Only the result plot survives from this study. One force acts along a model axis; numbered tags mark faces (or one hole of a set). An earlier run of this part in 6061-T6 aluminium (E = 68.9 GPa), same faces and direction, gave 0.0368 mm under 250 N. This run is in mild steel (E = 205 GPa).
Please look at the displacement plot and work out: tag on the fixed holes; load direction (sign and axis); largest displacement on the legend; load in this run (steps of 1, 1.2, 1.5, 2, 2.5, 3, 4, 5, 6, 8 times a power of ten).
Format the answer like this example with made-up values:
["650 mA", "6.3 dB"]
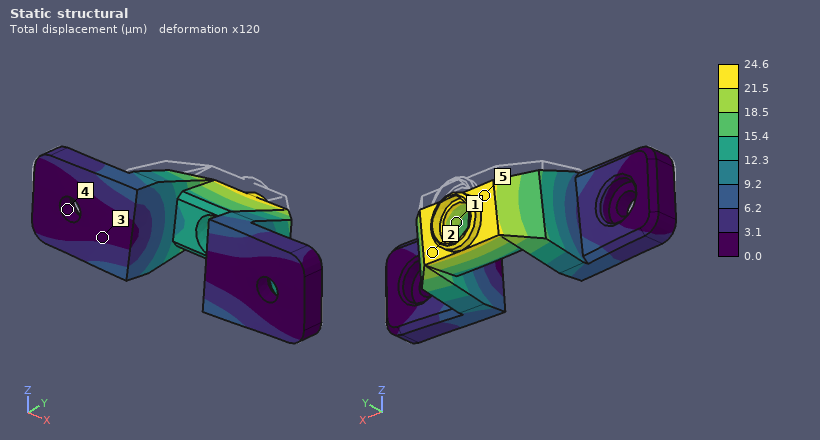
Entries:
["4", "-Z", "24.6 µm", "500 N"]
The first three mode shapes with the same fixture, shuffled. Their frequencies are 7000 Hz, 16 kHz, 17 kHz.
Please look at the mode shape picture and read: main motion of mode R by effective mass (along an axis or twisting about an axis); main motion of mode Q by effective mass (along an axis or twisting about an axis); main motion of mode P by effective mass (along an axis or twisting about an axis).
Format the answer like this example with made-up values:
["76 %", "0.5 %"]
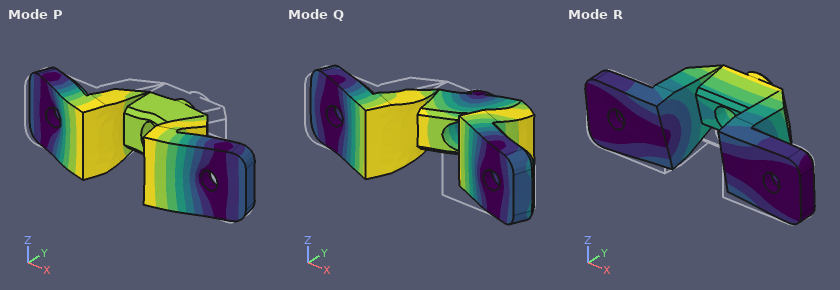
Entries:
["along Z", "along X", "along Y"]
